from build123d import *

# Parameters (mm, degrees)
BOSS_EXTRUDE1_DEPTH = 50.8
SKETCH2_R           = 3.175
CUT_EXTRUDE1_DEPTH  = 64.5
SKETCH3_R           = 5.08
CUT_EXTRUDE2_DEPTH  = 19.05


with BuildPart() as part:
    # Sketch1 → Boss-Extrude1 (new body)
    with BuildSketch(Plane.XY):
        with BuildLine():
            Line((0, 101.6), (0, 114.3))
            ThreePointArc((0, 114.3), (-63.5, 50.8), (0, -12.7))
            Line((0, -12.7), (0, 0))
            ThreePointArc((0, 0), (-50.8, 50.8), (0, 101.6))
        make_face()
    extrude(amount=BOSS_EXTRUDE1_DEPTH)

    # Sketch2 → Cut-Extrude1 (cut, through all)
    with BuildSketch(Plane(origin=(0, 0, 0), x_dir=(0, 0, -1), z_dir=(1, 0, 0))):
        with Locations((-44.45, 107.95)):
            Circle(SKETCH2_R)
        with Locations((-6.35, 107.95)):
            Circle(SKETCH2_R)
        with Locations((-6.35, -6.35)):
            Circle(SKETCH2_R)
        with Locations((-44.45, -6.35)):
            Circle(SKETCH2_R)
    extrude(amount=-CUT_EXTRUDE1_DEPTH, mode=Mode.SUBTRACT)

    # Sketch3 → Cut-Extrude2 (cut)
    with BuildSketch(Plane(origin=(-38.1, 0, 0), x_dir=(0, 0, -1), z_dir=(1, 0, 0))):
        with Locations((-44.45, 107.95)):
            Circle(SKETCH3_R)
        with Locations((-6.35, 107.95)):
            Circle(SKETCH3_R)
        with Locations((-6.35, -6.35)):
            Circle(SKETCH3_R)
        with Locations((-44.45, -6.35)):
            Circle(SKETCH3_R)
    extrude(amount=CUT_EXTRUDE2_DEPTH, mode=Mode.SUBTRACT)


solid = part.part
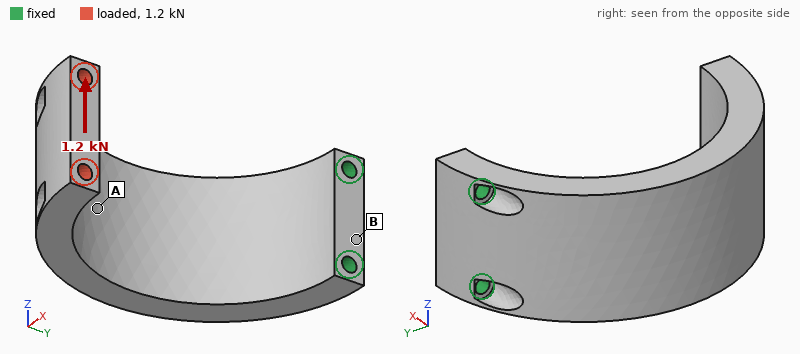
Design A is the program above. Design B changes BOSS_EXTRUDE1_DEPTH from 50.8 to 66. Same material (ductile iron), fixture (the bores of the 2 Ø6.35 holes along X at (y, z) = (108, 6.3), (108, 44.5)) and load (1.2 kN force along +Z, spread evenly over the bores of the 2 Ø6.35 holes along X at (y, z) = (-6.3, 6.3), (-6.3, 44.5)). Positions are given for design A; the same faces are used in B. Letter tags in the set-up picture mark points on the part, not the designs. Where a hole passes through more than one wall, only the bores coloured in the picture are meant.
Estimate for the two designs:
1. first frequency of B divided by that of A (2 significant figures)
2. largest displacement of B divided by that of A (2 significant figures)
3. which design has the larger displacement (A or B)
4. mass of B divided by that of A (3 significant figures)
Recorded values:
1.0
0.73
A
1.31
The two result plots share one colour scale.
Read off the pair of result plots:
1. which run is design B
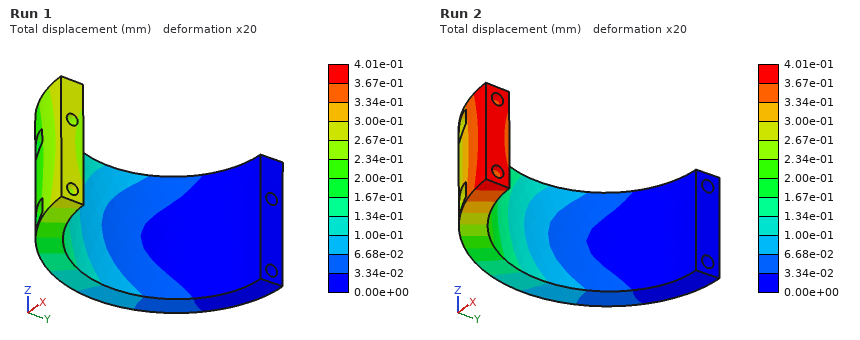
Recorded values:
Run 1
